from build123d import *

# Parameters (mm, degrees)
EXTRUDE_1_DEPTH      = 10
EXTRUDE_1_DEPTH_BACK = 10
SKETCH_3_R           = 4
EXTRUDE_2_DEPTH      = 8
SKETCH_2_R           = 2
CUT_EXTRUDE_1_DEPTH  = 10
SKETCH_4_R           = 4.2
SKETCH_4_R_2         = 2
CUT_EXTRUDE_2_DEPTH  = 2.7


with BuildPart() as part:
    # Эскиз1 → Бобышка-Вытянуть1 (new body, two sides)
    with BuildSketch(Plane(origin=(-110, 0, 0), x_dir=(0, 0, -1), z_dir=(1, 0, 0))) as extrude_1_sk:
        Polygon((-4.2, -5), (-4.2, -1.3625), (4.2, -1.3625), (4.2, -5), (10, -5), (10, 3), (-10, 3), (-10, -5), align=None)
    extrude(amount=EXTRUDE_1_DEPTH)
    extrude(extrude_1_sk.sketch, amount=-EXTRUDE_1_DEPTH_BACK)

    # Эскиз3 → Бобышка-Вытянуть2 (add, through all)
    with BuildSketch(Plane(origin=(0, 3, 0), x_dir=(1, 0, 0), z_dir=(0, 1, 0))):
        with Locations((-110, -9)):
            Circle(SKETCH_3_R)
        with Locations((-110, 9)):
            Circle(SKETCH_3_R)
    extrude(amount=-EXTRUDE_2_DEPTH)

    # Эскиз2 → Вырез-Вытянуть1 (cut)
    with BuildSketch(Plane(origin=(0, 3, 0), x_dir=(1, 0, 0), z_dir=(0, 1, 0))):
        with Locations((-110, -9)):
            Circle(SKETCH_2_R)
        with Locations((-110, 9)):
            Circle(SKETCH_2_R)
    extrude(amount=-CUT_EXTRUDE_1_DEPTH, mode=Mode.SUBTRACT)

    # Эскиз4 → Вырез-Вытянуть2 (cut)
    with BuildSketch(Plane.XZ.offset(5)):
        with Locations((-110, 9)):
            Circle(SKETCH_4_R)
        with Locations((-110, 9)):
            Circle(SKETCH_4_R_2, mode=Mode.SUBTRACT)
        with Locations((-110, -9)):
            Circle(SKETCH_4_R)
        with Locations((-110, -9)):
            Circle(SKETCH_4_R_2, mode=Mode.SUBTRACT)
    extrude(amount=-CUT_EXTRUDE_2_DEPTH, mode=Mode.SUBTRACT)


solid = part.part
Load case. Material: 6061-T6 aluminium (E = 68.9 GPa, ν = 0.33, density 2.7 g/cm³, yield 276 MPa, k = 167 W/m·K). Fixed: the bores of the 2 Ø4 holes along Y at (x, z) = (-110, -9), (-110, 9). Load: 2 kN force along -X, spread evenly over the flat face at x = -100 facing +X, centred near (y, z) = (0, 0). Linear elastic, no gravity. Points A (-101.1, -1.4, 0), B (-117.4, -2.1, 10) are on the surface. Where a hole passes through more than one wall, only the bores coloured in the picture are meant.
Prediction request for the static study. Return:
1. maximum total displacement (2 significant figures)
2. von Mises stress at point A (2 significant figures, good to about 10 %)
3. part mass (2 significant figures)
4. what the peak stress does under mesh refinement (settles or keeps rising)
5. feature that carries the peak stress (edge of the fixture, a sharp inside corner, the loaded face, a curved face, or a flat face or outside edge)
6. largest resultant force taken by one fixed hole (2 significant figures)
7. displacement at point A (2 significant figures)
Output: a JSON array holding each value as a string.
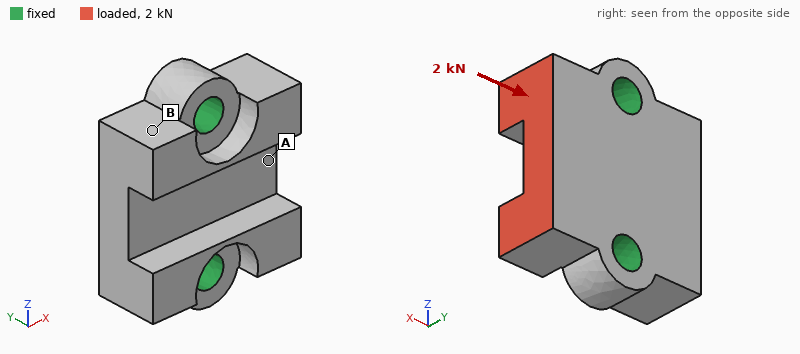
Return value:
["6.8 µm", "14 MPa", "6.6 g", "keeps rising", "a sharp inside corner", "1.0 kN", "4.4 µm"]
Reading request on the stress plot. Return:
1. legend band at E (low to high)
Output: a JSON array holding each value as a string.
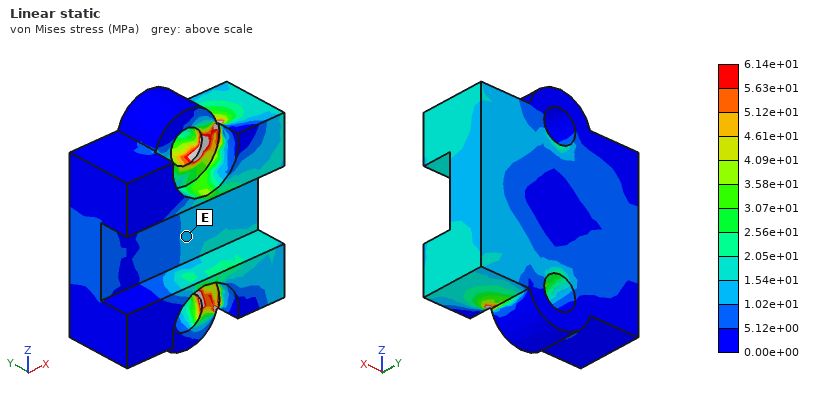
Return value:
["1.02e+01 to 1.54e+01 MPa"]
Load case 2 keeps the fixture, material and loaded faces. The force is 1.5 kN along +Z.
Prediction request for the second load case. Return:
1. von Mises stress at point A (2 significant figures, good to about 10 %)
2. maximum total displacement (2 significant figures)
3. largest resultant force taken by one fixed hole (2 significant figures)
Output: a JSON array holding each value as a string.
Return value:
["32 MPa", "11 µm", "1.0 kN"]
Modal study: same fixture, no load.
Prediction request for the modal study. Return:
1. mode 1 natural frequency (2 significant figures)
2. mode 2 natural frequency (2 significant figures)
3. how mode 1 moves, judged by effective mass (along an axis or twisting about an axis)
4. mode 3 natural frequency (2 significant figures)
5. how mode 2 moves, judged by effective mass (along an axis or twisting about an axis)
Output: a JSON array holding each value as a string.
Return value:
["30 kHz", "37 kHz", "twisting about Z", "44 kHz", "along Y"]
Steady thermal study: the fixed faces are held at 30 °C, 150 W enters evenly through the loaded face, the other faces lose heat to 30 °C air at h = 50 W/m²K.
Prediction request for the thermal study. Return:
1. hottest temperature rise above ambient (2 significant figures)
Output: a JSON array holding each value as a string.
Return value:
["78 K"]
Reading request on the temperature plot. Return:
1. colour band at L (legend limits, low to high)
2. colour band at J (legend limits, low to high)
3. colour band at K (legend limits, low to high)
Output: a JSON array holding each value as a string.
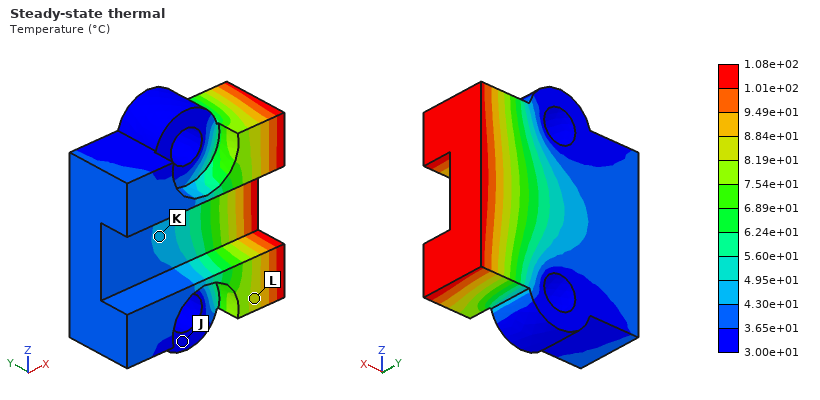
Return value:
["8.19e+01 to 8.84e+01 °C", "3.00e+01 to 3.65e+01 °C", "4.30e+01 to 4.95e+01 °C"]
